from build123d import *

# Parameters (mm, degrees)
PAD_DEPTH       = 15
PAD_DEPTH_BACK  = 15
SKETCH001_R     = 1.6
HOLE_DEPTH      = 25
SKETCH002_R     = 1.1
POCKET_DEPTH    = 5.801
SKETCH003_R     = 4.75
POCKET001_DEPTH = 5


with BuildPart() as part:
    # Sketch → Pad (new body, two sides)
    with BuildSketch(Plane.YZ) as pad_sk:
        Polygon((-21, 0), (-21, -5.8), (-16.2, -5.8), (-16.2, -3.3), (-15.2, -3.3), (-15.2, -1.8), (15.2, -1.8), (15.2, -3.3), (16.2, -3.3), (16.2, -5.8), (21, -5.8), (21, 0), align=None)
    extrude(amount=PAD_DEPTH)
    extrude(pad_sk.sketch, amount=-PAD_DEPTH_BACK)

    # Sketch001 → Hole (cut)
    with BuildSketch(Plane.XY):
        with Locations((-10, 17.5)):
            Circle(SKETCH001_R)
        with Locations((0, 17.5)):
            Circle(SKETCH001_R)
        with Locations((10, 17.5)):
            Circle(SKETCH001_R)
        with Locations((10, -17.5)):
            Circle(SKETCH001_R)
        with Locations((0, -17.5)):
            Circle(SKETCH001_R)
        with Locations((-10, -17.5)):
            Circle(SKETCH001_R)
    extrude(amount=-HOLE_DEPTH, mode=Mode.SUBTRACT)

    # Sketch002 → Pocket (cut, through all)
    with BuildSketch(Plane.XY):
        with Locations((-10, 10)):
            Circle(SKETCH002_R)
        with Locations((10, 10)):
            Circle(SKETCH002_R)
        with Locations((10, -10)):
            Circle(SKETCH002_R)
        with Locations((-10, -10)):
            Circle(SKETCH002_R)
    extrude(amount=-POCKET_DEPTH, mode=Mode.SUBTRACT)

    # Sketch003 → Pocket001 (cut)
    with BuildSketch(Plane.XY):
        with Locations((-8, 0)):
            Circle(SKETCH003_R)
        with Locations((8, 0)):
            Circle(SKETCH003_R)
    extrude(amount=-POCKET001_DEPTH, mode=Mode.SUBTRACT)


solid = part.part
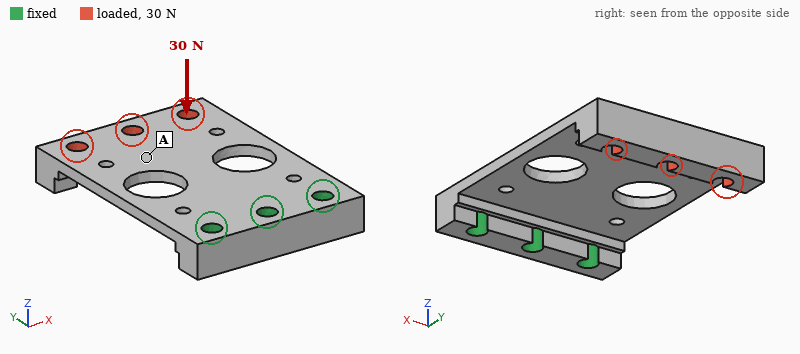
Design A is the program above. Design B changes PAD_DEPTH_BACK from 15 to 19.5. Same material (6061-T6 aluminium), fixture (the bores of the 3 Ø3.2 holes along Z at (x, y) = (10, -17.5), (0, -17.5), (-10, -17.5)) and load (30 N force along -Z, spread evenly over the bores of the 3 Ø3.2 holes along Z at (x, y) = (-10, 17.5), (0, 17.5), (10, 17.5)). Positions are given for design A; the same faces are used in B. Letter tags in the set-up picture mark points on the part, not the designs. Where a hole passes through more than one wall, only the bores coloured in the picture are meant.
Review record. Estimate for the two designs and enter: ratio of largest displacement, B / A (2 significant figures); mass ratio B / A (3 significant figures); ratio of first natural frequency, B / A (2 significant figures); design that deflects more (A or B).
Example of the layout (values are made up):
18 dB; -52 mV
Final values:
0.84; 1.18; 1.0; A
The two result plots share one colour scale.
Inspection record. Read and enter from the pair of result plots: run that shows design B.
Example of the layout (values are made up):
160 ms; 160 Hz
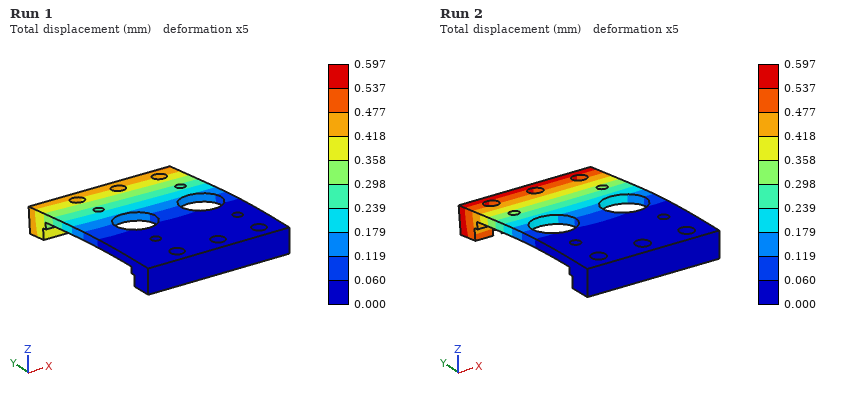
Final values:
Run 1
